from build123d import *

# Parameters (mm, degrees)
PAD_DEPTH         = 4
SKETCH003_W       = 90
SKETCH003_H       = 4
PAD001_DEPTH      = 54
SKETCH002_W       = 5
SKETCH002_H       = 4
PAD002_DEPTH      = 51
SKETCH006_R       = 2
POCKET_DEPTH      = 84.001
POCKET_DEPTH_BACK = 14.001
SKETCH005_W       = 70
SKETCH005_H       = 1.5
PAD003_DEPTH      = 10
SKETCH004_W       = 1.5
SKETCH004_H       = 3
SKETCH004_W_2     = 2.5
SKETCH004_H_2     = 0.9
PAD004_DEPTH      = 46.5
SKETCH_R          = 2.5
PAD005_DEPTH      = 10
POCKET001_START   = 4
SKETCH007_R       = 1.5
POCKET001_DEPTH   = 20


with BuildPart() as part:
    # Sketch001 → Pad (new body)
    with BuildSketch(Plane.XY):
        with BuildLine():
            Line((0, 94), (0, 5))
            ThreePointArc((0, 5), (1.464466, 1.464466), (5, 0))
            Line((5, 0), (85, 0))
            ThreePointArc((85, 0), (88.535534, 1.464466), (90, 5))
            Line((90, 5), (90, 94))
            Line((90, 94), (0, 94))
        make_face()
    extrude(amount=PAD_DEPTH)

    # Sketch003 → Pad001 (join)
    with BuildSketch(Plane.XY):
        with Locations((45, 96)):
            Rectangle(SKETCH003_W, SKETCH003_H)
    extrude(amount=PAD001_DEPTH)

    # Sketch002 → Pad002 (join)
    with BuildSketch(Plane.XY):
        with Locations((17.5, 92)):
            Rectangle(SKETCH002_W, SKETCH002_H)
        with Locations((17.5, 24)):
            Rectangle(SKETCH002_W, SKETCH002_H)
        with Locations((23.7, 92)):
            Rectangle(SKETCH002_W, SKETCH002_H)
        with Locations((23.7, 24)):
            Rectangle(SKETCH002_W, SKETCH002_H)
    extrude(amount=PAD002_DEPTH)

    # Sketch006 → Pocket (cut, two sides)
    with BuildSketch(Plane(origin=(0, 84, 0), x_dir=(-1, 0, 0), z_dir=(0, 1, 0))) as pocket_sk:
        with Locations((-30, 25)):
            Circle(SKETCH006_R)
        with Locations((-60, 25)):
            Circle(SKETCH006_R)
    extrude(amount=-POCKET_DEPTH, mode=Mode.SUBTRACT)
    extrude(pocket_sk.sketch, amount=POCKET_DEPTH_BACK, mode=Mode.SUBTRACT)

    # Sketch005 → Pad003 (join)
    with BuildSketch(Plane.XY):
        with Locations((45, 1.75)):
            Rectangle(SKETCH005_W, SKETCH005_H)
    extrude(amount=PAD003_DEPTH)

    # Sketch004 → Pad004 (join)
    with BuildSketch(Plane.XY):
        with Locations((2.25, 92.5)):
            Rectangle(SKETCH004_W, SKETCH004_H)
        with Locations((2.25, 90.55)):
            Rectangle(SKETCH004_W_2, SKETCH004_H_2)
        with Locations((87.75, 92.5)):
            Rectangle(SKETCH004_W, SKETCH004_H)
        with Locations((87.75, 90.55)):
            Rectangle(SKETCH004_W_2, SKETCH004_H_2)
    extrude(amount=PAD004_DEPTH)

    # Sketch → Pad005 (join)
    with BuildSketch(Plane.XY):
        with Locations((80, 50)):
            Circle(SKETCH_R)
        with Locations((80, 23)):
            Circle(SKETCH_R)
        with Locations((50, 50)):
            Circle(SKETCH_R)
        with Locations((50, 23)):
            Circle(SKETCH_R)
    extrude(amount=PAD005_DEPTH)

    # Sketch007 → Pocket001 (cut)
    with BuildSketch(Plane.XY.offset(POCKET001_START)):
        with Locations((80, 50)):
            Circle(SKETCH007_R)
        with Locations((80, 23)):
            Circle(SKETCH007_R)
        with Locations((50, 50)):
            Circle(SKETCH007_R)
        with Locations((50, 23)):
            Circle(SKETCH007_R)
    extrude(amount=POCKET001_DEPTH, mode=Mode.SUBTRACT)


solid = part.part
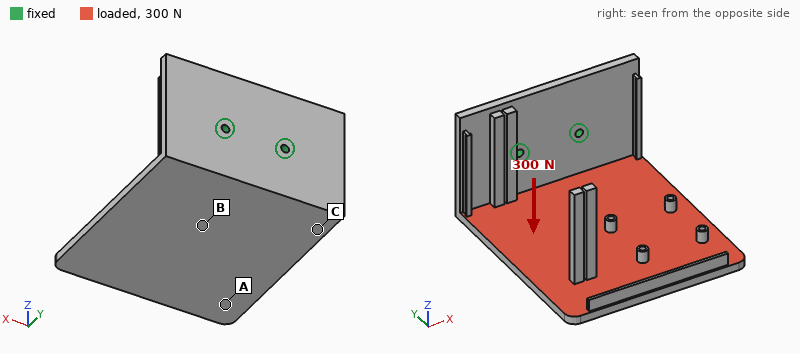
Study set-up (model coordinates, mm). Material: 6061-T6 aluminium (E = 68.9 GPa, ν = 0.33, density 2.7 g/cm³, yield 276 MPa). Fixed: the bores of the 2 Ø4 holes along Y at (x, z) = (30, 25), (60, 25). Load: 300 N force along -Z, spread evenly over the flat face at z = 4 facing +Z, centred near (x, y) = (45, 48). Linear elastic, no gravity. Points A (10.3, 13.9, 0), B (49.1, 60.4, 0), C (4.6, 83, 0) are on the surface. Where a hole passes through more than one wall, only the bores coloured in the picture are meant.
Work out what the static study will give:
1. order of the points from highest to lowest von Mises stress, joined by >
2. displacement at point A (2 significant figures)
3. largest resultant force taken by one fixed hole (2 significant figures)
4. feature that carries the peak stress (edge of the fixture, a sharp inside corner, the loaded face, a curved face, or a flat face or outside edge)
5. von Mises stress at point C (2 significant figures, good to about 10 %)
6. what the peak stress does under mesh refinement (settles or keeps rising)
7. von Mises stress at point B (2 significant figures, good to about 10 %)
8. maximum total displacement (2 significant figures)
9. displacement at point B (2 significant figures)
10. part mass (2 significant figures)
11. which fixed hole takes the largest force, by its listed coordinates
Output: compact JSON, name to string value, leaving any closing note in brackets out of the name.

{"order of the points from highest to lowest von Mises stress, joined by >": "C > B > A", "displacement at point A": "1.2 mm", "largest resultant force taken by one fixed hole": "170 N", "feature that carries the peak stress": "edge of the fixture", "von Mises stress at point C": "49 MPa", "what the peak stress does under mesh refinement": "keeps rising", "von Mises stress at point B": "21 MPa", "maximum total displacement": "1.6 mm", "displacement at point B": "0.45 mm", "part mass": "160 g", "which fixed hole takes the largest force, by its listed coordinates": "(60, 25)"}
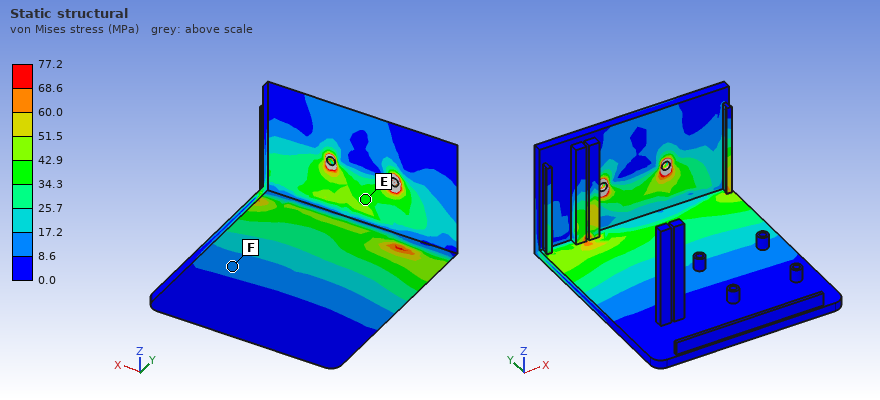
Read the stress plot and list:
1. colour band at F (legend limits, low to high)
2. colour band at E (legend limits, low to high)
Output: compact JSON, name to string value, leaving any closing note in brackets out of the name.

{"colour band at F": "8.6 to 17.2 MPa", "colour band at E": "34.3 to 42.9 MPa"}
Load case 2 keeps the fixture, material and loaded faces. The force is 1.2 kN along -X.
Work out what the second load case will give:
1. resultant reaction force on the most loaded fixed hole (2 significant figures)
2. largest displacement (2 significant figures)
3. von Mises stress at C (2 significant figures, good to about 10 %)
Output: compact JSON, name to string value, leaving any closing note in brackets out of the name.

{"resultant reaction force on the most loaded fixed hole": "1.8 kN", "largest displacement": "1.2 mm", "von Mises stress at C": "41 MPa"}
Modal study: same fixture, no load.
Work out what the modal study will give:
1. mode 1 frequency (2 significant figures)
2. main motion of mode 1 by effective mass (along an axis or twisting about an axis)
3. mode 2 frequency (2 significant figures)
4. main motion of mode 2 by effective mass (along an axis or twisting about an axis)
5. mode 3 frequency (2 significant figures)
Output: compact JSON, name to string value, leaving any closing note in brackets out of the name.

{"mode 1 frequency": "260 Hz", "main motion of mode 1 by effective mass": "along Z", "mode 2 frequency": "560 Hz", "main motion of mode 2 by effective mass": "along X", "mode 3 frequency": "870 Hz"}
